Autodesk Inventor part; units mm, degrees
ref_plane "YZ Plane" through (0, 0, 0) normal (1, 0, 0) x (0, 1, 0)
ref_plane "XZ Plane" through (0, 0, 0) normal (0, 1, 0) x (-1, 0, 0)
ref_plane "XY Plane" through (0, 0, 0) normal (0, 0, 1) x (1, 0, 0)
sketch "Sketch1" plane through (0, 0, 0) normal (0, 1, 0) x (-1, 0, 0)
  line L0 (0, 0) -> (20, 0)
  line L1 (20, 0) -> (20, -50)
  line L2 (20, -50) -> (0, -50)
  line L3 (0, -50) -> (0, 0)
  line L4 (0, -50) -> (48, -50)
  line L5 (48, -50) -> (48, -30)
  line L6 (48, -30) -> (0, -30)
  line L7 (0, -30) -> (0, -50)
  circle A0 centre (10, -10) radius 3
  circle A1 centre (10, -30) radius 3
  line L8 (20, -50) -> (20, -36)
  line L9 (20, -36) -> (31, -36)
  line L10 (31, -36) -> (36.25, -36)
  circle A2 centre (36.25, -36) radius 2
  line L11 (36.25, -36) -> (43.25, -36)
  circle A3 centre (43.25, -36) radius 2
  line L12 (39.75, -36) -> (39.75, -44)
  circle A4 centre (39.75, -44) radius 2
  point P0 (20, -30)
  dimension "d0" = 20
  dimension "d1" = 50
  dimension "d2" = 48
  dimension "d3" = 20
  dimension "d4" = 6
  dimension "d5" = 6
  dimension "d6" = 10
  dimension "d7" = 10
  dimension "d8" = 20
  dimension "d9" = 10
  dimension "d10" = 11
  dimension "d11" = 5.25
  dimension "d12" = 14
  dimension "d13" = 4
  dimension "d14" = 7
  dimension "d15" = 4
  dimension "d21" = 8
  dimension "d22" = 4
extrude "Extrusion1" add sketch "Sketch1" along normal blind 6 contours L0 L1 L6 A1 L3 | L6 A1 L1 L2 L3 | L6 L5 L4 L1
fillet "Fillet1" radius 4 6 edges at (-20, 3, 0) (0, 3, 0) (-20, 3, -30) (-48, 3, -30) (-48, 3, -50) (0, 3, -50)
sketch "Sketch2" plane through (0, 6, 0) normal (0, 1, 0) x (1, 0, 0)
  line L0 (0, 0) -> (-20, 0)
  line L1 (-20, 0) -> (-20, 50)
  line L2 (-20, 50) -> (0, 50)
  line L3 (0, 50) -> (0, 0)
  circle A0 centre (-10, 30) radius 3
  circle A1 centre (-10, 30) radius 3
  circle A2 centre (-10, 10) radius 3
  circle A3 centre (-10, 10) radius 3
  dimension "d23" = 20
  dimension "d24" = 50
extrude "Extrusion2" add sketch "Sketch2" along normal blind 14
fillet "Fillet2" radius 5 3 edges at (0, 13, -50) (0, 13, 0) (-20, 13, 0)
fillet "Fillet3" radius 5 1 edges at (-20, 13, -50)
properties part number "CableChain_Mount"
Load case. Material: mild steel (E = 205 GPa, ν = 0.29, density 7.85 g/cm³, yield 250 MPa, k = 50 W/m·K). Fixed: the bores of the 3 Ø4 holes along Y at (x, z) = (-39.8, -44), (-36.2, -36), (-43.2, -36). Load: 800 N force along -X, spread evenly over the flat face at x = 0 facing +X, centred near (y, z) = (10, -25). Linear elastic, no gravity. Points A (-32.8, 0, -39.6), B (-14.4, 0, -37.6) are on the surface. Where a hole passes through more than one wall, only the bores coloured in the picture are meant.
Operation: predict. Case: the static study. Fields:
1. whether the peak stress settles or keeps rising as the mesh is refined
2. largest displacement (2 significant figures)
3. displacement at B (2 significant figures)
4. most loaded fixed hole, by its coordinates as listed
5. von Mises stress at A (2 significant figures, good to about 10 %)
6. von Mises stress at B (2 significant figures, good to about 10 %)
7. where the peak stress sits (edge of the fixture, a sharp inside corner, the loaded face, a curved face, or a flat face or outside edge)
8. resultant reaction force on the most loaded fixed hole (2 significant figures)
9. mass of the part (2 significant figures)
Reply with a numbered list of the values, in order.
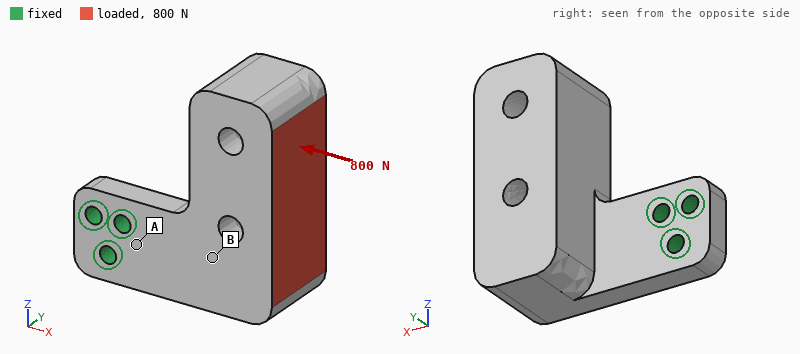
1. keeps rising
2. 55 µm
3. 18 µm
4. (-36.2, -36)
5. 38 MPa
6. 11 MPa
7. edge of the fixture
8. 1.2 kN
9. 170 g
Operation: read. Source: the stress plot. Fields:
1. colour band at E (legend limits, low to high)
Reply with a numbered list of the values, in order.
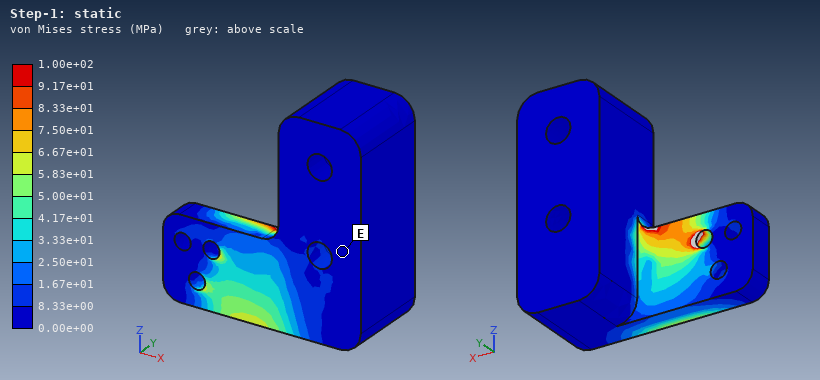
1. 0.00e+00 to 8.33e+00 MPa
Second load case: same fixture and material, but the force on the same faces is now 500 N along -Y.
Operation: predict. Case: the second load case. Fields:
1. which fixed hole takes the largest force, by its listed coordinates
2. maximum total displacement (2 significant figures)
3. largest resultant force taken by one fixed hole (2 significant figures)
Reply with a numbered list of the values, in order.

1. (-36.2, -36)
2. 0.14 mm
3. 1.2 kN
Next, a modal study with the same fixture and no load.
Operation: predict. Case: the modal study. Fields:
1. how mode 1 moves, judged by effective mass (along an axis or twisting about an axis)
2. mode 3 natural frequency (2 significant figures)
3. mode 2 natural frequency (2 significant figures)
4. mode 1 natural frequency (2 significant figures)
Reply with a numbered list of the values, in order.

1. along Y
2. 3000 Hz
3. 2000 Hz
4. 1100 Hz
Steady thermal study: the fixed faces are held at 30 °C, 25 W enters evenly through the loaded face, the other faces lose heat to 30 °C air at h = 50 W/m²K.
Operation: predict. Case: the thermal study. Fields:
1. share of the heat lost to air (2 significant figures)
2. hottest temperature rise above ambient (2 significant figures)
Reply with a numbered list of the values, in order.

1. 48 %
2. 61 K
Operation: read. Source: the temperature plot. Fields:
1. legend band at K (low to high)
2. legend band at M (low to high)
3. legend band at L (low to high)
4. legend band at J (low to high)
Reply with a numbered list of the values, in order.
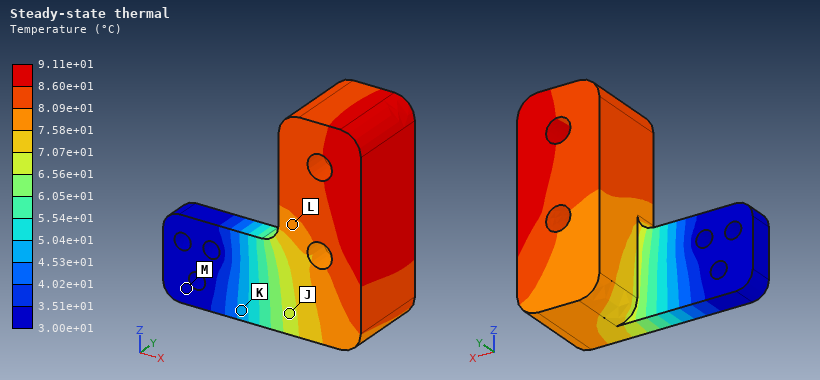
1. 4.53e+01 to 5.04e+01 °C
2. 3.00e+01 to 3.51e+01 °C
3. 7.58e+01 to 8.09e+01 °C
4. 6.56e+01 to 7.07e+01 °C
